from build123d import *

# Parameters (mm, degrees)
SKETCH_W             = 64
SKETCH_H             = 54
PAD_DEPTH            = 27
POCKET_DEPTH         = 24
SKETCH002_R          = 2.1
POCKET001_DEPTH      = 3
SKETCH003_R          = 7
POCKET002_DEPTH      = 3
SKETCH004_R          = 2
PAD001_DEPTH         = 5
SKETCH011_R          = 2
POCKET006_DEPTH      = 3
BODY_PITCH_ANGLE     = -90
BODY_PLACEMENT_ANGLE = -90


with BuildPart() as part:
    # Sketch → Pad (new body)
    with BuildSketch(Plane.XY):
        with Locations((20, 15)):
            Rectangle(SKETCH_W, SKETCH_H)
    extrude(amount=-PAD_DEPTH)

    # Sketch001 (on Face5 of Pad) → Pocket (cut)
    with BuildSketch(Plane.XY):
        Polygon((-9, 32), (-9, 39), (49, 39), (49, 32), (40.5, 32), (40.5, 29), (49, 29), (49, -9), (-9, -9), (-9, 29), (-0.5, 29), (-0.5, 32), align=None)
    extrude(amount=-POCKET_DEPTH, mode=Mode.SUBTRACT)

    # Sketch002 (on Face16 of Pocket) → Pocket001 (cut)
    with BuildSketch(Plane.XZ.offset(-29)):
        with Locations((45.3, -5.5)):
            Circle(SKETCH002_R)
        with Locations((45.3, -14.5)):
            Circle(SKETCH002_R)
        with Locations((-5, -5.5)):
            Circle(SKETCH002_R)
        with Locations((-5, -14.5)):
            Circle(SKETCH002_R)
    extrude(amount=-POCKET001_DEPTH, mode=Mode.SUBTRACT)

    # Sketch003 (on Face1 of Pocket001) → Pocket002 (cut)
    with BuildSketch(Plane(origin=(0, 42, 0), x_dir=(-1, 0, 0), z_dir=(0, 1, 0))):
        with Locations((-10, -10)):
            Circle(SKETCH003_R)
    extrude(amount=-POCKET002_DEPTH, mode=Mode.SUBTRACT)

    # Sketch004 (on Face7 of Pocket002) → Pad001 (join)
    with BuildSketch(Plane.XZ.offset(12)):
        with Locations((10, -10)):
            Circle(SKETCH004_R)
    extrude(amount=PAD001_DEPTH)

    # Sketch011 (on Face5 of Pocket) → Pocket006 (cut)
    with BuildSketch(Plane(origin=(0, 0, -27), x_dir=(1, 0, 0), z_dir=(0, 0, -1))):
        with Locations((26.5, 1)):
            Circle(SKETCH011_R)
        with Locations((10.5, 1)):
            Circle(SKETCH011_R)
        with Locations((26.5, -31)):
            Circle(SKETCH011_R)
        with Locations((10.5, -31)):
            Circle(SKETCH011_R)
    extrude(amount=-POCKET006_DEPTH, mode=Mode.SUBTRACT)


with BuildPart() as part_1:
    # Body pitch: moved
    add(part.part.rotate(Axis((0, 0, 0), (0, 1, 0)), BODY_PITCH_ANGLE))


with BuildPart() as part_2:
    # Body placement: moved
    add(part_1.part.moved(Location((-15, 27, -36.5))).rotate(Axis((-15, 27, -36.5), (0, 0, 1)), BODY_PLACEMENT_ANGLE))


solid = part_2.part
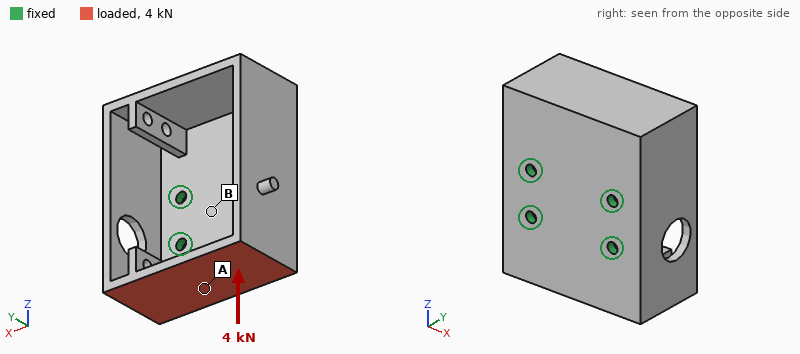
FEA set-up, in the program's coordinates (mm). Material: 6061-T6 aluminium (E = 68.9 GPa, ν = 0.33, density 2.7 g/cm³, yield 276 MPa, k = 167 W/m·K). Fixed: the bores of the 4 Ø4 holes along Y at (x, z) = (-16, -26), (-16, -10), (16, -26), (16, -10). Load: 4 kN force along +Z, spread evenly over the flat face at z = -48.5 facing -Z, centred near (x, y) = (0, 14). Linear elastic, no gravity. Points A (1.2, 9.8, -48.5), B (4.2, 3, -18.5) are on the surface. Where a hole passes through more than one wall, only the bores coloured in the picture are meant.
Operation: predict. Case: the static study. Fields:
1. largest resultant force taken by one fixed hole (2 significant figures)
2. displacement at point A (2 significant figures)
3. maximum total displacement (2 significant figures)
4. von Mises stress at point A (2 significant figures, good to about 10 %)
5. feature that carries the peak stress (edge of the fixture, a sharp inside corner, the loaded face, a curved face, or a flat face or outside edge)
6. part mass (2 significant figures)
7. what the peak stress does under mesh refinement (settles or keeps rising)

1.7 kN
0.23 mm
0.49 mm
56 MPa
edge of the fixture
73 g
keeps rising
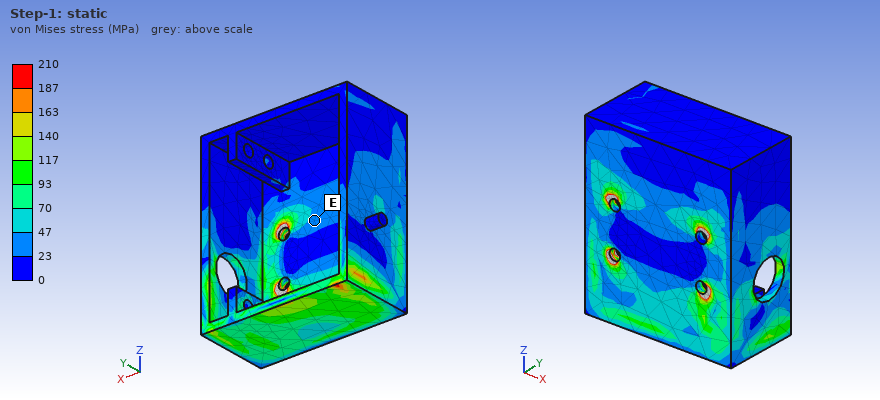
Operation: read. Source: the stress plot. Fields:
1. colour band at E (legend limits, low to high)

23 to 47 MPa
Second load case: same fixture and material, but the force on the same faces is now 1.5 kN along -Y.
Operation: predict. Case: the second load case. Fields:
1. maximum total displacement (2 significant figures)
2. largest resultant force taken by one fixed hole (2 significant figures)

0.21 mm
1.4 kN
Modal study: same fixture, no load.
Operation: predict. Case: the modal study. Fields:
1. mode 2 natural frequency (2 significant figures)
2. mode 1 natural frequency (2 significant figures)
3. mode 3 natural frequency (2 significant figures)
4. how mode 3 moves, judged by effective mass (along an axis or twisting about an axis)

2800 Hz
2600 Hz
3900 Hz
along X
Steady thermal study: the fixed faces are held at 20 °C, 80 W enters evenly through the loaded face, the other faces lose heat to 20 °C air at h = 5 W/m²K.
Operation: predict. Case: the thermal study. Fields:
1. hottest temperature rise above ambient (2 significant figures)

67 K
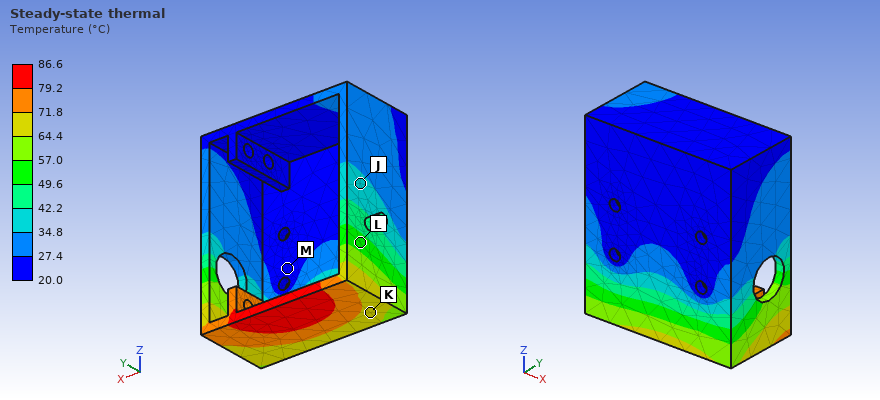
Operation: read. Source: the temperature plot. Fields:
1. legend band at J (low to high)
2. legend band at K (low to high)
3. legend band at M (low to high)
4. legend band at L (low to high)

34.8 to 42.2 °C
64.4 to 71.8 °C
20.0 to 27.4 °C
49.6 to 57.0 °C
